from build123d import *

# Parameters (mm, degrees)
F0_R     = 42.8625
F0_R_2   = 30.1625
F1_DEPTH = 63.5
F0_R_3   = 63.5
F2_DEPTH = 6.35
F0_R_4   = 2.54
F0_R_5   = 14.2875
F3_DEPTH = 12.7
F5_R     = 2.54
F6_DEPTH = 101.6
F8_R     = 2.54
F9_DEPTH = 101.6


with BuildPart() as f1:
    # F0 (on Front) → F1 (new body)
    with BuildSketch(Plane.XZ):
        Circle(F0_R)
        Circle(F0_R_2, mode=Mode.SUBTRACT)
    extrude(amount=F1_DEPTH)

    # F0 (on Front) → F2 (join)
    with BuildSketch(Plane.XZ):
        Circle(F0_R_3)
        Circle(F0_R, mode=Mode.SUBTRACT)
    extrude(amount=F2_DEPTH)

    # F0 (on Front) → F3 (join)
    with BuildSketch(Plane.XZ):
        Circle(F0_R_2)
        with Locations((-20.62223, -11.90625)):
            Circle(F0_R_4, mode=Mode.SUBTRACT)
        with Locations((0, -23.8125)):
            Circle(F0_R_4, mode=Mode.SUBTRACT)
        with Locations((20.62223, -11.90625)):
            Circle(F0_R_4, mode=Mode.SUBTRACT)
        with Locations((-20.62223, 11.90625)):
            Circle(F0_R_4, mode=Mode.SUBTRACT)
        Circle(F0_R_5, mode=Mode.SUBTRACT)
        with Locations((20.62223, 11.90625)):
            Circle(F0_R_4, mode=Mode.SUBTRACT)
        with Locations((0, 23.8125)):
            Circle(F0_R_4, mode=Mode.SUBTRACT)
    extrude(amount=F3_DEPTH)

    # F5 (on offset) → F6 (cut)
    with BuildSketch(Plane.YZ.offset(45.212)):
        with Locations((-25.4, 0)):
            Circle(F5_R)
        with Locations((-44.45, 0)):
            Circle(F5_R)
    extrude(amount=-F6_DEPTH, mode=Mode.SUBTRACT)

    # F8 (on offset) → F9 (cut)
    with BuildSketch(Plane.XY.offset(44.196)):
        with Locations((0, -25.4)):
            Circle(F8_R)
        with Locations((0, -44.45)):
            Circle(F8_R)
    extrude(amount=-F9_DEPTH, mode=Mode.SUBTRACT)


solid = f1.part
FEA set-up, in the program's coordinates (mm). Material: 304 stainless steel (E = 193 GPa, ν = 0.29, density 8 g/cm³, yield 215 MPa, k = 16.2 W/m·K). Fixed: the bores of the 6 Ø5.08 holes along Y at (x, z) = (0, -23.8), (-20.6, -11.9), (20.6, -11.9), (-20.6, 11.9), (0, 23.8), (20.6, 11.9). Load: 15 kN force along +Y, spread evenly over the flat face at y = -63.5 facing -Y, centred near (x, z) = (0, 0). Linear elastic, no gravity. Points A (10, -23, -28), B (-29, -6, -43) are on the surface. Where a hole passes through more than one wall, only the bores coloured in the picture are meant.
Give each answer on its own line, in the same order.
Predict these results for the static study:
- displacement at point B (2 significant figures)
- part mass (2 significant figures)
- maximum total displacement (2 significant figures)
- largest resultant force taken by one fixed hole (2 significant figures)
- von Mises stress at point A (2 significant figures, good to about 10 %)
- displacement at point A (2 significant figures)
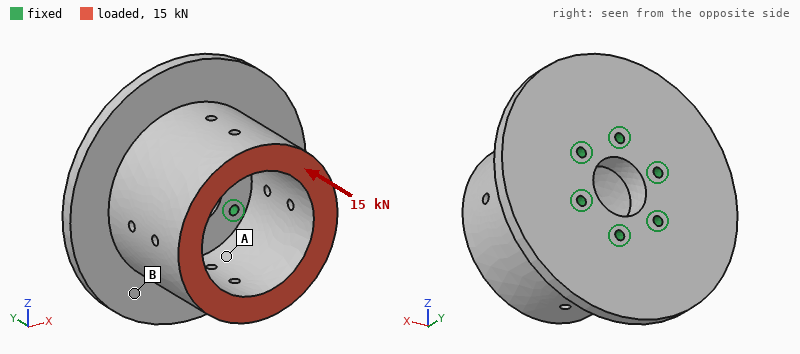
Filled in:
3.3 µm
2.0 kg
4.2 µm
2.5 kN
11 MPa
2.4 µm
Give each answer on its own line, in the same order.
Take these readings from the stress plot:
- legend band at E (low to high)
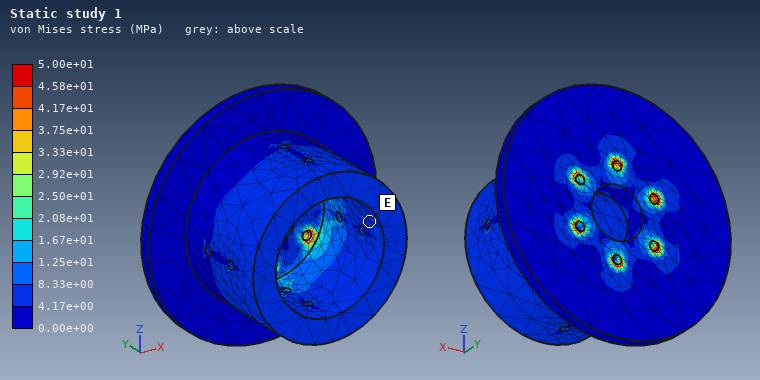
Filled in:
4.17e+00 to 8.33e+00 MPa
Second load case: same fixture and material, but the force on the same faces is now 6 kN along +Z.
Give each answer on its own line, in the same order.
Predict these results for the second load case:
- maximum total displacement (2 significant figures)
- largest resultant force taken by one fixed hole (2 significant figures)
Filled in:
14 µm
3.4 kN
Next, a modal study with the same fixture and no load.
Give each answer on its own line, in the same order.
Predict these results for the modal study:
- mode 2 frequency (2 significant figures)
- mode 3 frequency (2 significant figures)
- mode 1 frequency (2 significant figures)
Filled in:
4300 Hz
6300 Hz
4300 Hz
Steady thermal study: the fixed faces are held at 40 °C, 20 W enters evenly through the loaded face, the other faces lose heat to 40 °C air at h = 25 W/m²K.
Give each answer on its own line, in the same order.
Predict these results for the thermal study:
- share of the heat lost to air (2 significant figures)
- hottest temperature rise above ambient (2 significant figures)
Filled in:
46 %
22 K
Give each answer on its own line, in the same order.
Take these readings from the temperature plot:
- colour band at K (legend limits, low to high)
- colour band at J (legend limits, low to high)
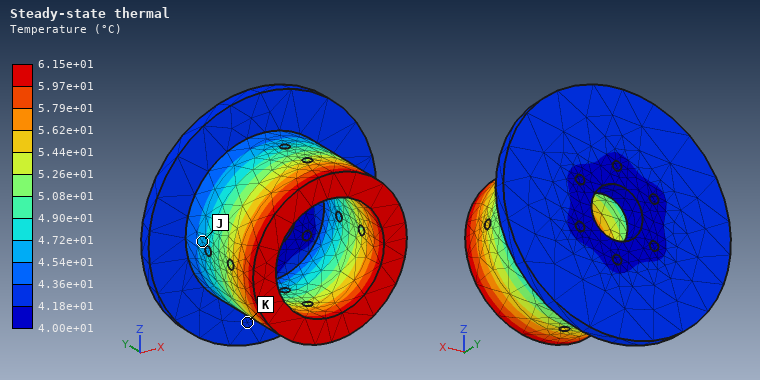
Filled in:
4.18e+01 to 4.36e+01 °C
4.54e+01 to 4.72e+01 °C
